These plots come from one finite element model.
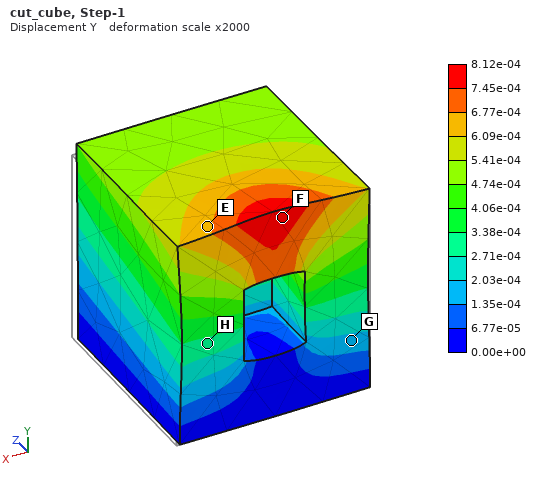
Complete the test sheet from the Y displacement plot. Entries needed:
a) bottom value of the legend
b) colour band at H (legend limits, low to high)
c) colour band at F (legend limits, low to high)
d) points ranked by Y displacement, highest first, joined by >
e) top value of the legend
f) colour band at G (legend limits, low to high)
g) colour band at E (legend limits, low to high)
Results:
0.00e+00
2.71e-04 to 3.38e-04
7.45e-04 to 8.12e-04
F > E > H > G
8.12e-04
1.35e-04 to 2.03e-04
6.09e-04 to 6.77e-04
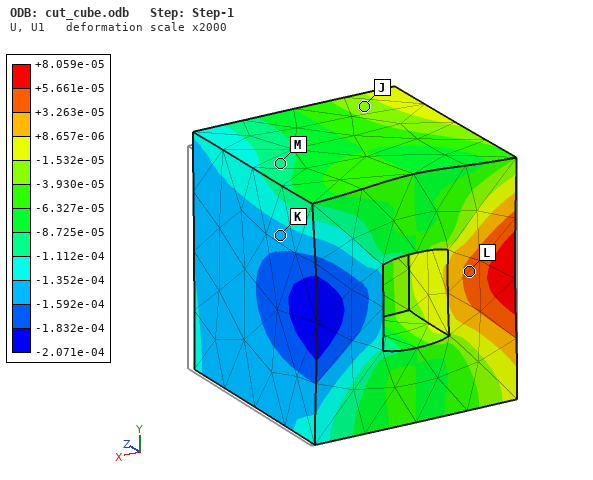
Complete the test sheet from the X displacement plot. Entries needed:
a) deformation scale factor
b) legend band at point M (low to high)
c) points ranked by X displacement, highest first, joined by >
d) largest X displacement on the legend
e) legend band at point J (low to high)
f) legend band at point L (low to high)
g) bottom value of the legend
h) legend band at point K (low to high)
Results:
2000
-1.112e-04 to -8.725e-05
L > J > M > K
+8.059e-05
-3.930e-05 to -1.532e-05
+3.263e-05 to +5.661e-05
-2.071e-04
-1.592e-04 to -1.352e-04
